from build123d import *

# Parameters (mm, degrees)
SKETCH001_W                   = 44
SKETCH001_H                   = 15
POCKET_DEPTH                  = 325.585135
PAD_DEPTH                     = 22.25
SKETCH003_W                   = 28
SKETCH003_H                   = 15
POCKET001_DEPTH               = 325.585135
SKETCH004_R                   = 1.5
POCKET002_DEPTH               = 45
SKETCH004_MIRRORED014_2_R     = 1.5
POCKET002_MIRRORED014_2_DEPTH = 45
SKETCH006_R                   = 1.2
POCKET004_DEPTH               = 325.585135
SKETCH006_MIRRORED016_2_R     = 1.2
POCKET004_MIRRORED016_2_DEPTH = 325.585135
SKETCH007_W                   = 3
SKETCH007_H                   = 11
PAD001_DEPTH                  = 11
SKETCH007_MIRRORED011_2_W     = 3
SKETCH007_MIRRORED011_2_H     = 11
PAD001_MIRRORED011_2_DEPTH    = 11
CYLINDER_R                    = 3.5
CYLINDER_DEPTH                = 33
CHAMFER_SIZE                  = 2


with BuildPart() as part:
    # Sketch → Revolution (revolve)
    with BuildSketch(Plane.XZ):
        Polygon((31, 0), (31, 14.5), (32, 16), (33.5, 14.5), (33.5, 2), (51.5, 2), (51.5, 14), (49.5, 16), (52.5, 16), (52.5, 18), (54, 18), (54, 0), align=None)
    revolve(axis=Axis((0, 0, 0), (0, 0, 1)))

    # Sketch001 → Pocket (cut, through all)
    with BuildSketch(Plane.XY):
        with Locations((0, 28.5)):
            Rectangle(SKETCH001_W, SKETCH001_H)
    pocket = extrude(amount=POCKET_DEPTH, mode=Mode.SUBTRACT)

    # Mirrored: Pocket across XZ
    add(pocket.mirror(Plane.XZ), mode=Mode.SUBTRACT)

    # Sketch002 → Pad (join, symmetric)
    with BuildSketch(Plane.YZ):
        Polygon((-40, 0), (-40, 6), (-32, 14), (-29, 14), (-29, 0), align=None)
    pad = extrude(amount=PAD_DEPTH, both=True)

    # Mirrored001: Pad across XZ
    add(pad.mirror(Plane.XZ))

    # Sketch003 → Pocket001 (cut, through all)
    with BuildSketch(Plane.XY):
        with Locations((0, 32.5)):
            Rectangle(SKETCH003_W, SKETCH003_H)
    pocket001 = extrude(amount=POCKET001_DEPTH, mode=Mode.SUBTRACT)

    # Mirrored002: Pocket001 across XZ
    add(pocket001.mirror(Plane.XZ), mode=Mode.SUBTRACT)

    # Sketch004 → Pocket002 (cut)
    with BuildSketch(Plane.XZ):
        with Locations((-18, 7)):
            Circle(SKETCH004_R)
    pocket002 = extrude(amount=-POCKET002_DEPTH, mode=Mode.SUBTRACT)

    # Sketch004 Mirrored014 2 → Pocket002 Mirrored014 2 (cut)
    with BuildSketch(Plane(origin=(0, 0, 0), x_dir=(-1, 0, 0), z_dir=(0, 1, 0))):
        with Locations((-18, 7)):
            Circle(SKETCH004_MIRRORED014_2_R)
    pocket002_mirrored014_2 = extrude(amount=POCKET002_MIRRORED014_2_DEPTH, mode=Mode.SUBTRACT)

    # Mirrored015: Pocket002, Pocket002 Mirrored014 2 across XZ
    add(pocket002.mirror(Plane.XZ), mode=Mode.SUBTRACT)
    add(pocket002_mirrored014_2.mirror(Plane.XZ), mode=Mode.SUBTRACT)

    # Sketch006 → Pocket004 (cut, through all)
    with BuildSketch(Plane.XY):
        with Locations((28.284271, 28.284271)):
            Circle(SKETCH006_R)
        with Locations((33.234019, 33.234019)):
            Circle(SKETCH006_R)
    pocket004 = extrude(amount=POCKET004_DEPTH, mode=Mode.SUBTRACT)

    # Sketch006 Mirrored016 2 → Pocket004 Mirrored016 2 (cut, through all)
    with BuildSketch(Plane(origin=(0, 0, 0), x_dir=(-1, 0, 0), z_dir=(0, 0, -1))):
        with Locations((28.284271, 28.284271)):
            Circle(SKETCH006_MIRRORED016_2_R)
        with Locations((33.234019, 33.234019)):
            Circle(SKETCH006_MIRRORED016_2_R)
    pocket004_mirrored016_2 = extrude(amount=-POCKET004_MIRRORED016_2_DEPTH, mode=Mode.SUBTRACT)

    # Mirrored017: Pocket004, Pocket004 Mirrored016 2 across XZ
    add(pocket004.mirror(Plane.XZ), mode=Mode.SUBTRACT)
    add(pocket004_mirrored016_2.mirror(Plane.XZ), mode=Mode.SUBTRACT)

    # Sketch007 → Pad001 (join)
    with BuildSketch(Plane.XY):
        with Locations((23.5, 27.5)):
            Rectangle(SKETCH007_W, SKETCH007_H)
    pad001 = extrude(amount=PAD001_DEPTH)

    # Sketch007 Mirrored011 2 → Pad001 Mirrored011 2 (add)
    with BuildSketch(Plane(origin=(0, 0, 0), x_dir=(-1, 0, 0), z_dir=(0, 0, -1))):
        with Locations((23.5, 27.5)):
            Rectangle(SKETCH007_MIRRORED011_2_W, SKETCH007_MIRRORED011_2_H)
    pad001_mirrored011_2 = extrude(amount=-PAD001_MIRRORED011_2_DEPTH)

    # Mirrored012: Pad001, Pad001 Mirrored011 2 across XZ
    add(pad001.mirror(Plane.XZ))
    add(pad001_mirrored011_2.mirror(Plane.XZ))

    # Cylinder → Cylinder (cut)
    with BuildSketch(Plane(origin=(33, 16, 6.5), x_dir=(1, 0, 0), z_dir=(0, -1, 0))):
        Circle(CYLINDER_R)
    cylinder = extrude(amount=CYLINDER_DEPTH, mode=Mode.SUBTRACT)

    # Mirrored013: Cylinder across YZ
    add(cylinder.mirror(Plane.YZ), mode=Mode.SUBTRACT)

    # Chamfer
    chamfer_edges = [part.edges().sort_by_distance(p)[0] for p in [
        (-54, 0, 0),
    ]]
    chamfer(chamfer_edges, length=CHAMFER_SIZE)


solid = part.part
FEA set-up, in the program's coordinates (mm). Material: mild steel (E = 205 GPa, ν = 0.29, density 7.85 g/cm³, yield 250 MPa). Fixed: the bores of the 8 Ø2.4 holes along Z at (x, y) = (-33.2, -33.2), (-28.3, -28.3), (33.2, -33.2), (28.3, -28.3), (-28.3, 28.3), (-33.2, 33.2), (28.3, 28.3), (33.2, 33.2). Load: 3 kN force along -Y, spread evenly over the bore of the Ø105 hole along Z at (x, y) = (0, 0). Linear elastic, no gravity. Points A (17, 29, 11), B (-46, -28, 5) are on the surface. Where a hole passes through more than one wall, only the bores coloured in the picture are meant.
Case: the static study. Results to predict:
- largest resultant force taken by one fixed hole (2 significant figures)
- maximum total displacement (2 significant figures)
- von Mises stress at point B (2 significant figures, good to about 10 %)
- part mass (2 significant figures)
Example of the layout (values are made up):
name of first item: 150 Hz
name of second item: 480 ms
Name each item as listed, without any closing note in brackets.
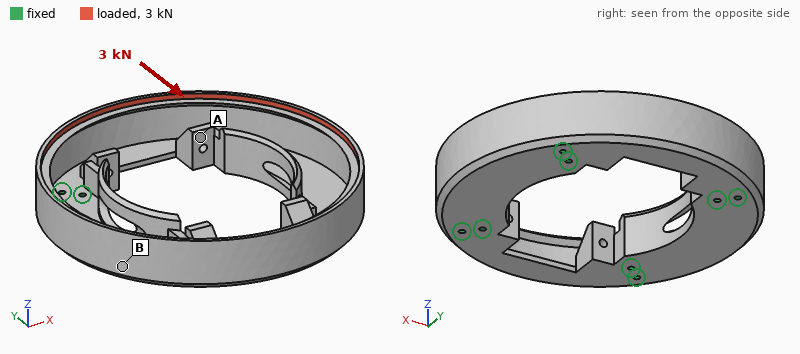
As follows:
largest resultant force taken by one fixed hole: 750 N
maximum total displacement: 38 µm
von Mises stress at point B: 11 MPa
part mass: 240 g
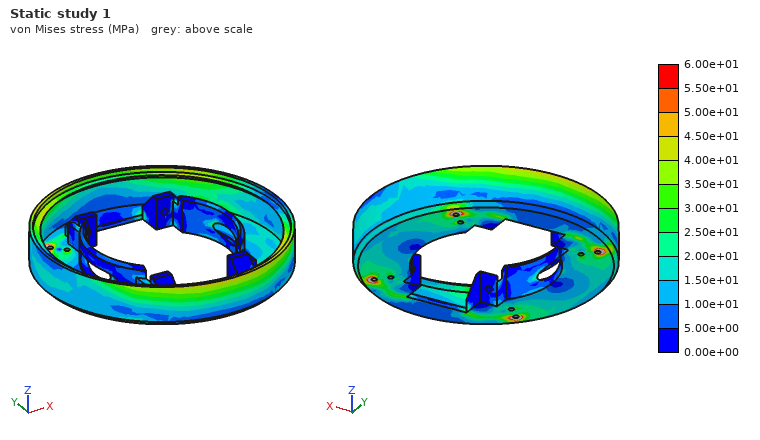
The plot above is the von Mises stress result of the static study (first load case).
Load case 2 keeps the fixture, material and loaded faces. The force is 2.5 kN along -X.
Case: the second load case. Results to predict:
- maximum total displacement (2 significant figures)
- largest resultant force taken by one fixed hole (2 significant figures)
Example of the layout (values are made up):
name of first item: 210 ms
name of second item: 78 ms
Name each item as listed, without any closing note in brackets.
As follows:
maximum total displacement: 36 µm
largest resultant force taken by one fixed hole: 720 N
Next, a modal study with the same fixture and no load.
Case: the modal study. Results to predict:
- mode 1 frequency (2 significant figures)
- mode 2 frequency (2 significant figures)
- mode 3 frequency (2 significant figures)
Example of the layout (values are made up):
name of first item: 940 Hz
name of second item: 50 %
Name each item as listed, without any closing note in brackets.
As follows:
mode 1 frequency: 1900 Hz
mode 2 frequency: 3600 Hz
mode 3 frequency: 3900 Hz
